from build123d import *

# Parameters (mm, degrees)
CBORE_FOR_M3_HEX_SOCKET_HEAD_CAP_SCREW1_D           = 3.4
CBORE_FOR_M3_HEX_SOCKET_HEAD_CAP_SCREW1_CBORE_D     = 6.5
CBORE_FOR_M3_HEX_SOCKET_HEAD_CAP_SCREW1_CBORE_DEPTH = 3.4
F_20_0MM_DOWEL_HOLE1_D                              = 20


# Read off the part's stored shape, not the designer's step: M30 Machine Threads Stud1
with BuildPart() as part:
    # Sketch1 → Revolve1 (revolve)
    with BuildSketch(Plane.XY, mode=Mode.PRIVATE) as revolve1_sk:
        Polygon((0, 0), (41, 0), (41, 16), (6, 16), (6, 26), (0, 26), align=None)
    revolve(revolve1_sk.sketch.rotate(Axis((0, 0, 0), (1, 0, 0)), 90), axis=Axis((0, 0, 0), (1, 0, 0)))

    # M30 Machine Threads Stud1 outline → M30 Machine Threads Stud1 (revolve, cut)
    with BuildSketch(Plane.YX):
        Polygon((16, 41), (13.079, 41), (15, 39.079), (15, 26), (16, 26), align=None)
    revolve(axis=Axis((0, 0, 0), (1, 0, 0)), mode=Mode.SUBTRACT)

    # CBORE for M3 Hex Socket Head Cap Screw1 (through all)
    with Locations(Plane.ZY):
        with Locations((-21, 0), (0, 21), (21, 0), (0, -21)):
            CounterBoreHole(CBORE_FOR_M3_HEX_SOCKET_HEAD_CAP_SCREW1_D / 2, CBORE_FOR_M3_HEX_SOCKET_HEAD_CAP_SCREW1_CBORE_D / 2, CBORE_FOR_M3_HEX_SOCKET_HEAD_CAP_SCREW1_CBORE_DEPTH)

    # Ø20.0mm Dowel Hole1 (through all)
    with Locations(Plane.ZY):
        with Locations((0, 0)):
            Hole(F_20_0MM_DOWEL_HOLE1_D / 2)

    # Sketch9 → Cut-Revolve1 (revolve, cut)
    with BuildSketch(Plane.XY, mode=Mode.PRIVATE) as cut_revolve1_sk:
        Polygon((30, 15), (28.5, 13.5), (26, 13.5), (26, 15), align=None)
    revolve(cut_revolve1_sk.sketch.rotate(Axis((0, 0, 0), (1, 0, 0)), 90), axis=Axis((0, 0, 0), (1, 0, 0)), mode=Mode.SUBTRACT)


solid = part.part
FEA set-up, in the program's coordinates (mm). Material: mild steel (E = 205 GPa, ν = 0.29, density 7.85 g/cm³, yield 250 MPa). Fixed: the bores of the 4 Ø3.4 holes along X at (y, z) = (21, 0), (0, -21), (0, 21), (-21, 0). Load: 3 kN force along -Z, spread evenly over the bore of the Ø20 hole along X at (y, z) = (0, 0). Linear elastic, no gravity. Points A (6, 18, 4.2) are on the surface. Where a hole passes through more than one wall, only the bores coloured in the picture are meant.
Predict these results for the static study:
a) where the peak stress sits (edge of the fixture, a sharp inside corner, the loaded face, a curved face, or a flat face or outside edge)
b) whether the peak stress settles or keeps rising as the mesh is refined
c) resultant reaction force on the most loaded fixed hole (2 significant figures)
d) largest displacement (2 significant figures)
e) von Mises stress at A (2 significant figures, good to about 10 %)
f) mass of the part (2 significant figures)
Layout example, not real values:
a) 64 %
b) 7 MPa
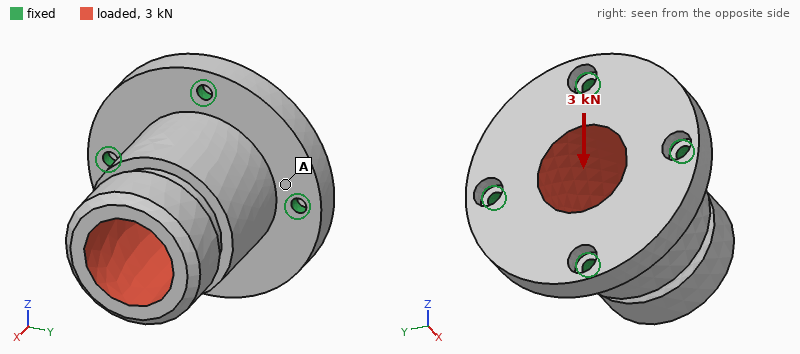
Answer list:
a) edge of the fixture
b) keeps rising
c) 1.3 kN
d) 13 µm
e) 20 MPa
f) 200 g
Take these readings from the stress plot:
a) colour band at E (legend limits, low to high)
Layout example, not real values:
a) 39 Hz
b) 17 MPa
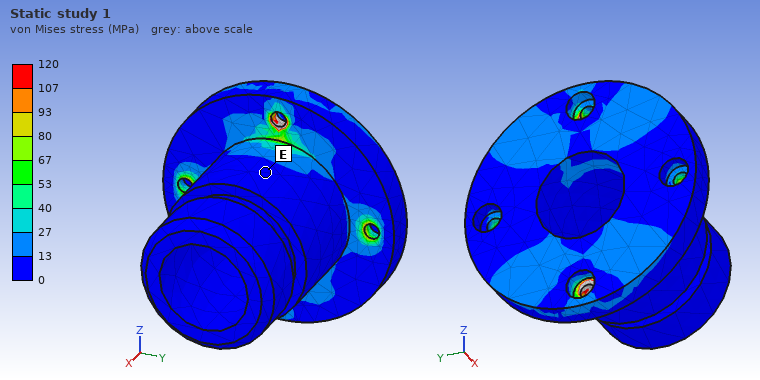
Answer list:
a) 0 to 13 MPa
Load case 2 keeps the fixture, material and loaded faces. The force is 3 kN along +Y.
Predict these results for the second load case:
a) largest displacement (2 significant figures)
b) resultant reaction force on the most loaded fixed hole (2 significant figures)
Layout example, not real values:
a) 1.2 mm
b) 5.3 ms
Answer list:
a) 13 µm
b) 1.3 kN
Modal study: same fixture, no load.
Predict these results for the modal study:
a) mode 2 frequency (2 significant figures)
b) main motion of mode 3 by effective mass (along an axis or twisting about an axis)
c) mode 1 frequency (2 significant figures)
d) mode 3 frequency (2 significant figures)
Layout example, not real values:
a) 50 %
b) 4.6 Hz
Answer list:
a) 7800 Hz
b) along X
c) 7800 Hz
d) 13 kHz
